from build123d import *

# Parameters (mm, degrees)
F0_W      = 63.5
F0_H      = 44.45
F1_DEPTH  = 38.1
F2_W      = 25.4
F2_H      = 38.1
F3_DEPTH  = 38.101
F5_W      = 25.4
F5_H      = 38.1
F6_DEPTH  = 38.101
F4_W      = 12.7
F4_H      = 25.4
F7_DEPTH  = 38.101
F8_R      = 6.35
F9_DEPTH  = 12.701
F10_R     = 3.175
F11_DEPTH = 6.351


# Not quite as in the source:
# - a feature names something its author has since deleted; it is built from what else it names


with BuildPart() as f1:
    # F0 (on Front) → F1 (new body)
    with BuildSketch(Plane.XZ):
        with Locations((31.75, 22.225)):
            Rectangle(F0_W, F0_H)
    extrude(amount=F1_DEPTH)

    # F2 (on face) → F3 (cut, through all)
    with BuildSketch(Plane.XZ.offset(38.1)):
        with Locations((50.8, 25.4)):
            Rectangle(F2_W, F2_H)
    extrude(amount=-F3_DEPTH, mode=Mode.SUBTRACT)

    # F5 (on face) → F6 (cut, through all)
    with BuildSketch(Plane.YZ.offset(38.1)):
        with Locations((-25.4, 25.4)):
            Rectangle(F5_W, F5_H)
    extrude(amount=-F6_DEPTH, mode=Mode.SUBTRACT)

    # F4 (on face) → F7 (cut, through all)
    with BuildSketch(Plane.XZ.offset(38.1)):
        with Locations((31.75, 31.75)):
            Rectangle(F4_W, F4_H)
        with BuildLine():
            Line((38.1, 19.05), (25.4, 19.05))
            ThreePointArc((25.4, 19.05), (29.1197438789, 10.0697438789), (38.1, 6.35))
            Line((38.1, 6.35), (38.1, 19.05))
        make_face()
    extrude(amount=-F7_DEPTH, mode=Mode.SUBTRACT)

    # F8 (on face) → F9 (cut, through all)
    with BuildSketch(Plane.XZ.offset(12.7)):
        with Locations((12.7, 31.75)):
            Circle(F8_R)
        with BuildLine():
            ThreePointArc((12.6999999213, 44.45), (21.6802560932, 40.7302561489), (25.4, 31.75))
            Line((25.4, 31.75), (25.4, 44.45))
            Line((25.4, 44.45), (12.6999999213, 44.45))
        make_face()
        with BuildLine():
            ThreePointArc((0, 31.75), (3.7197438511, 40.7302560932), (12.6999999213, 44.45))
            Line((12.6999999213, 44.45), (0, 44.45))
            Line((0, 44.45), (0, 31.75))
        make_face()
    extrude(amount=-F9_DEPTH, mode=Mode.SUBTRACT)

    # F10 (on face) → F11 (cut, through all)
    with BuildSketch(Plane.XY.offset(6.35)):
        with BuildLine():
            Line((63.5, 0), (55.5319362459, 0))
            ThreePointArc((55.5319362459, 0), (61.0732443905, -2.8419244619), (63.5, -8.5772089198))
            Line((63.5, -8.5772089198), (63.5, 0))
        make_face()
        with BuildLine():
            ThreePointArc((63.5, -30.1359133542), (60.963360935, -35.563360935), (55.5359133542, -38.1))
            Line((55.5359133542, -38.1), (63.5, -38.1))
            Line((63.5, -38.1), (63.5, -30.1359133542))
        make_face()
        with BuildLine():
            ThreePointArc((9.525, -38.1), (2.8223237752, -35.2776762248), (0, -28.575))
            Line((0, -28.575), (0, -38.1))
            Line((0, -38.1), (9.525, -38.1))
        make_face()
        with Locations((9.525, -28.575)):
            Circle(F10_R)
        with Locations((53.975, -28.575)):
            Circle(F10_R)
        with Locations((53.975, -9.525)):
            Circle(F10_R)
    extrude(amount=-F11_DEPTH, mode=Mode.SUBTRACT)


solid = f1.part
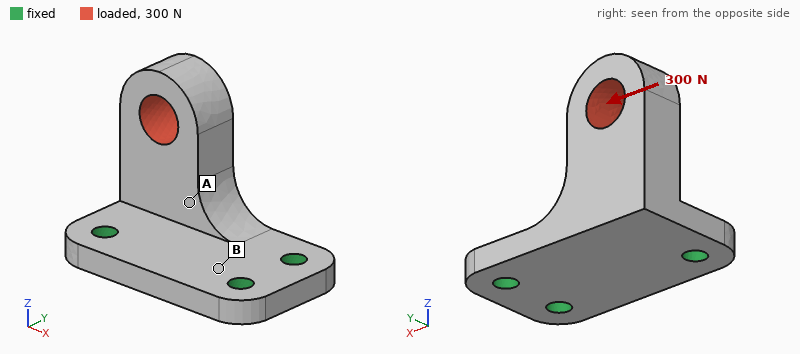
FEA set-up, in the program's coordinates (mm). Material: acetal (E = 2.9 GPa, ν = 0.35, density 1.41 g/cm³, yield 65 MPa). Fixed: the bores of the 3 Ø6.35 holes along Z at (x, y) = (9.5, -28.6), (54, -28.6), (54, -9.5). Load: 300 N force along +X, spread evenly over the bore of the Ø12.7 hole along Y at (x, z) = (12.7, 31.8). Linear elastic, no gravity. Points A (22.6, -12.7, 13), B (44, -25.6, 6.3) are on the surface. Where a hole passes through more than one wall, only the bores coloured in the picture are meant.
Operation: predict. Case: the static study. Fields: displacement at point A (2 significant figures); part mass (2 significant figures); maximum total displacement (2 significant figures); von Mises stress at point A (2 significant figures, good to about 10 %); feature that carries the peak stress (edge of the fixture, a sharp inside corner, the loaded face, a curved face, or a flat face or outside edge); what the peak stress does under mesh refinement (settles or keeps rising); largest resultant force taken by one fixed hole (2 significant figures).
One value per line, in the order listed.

0.16 mm
35 g
0.79 mm
6.6 MPa
edge of the fixture
keeps rising
230 N
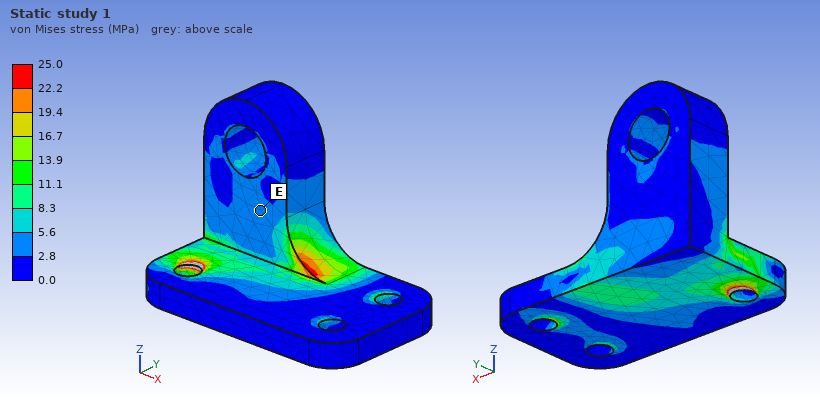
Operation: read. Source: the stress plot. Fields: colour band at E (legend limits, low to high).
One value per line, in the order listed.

2.8 to 5.6 MPa
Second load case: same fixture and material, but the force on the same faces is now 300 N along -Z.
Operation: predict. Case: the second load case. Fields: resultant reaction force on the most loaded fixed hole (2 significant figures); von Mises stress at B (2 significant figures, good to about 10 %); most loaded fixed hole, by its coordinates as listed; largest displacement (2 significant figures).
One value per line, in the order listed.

240 N
3.4 MPa
(9.5, -28.6)
0.89 mm
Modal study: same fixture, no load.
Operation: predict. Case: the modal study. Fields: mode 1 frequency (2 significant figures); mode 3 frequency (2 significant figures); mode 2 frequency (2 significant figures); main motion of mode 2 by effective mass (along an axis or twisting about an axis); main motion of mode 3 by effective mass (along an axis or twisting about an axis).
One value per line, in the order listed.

680 Hz
2200 Hz
1400 Hz
along X
along Z
